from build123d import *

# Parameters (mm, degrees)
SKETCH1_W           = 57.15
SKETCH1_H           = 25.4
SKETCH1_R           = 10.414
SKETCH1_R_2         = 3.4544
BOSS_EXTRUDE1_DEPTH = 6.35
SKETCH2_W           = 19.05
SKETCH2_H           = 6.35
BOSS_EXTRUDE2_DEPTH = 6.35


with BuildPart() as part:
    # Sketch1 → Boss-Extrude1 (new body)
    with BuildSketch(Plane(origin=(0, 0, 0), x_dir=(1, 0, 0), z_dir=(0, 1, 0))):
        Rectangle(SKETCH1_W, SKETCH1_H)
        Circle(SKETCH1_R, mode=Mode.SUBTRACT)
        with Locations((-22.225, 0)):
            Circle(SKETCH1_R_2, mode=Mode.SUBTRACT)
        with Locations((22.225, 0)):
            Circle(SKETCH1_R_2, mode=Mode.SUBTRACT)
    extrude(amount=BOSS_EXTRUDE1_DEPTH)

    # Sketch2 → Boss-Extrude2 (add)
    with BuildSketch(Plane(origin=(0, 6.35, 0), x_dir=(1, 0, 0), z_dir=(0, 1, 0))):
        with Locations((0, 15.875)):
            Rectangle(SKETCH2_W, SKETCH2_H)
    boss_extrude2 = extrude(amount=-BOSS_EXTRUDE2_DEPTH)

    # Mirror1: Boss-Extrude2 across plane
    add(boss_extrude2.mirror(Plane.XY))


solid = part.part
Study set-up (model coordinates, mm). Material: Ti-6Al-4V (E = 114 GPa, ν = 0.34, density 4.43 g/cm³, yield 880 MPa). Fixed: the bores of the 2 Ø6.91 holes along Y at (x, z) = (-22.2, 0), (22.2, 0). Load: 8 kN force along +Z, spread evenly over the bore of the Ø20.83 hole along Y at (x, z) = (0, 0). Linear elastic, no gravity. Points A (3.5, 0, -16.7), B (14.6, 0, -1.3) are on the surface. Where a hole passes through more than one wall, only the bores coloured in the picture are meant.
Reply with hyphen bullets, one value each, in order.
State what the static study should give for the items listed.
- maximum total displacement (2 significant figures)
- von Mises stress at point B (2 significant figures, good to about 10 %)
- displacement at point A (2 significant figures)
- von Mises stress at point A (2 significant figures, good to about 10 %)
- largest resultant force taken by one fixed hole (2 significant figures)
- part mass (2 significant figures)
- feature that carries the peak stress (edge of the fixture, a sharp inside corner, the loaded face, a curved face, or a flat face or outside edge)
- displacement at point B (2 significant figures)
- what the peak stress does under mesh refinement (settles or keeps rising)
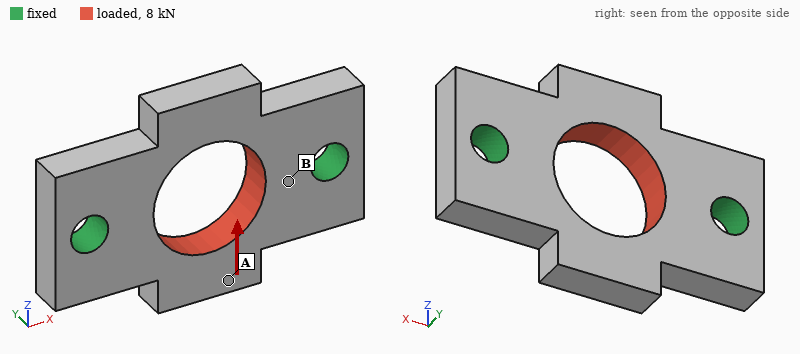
- 14 µm
- 59 MPa
- 13 µm
- 25 MPa
- 4.0 kN
- 36 g
- edge of the fixture
- 6.2 µm
- keeps rising
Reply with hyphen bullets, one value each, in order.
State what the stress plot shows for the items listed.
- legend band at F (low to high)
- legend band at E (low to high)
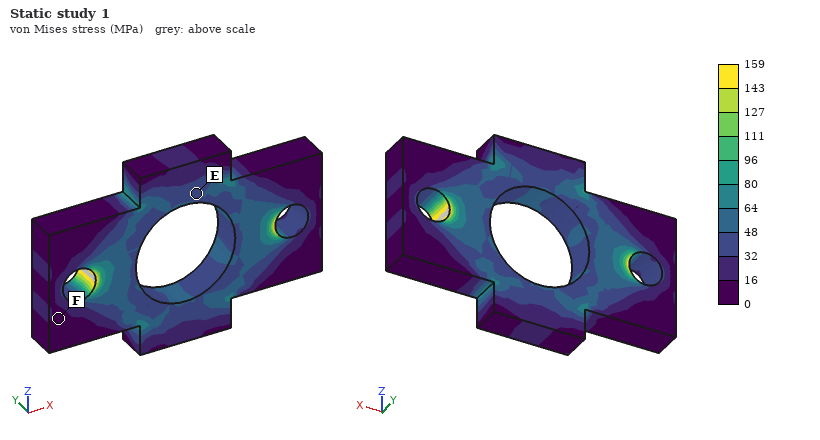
- 0 to 16 MPa
- 32 to 48 MPa
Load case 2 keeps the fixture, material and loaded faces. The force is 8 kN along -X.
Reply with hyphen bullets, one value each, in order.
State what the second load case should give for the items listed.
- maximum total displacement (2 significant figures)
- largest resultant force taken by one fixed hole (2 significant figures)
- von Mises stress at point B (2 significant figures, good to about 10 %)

- 7.4 µm
- 4.0 kN
- 35 MPa
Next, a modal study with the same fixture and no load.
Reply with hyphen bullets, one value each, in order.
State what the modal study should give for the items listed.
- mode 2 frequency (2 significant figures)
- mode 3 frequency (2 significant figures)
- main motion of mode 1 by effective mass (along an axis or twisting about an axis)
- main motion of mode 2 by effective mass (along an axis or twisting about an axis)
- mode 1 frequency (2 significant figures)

- 12 kHz
- 27 kHz
- twisting about X
- along Y
- 11 kHz
